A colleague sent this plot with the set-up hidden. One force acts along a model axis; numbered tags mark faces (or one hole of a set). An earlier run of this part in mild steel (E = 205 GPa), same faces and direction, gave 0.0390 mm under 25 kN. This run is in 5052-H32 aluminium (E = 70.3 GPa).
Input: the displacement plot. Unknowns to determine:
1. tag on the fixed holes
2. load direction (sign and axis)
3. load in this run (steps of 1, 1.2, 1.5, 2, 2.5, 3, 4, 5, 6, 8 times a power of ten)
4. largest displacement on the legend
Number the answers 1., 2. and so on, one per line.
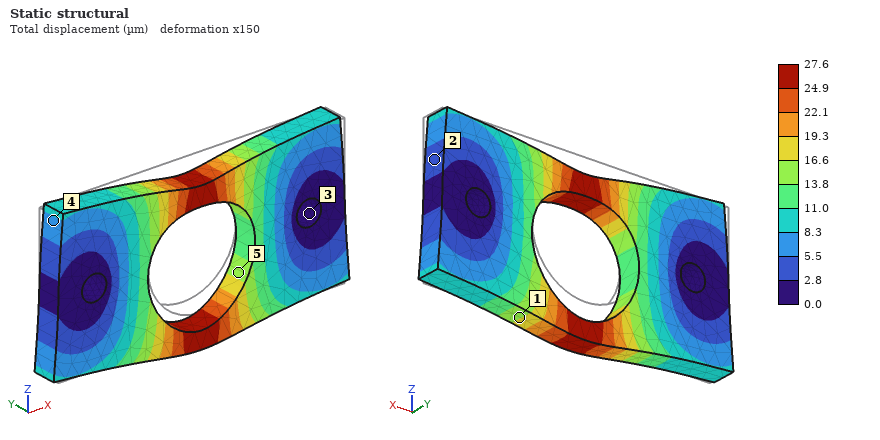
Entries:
1. 3
2. -Z
3. 6 kN
4. 27.6 µm
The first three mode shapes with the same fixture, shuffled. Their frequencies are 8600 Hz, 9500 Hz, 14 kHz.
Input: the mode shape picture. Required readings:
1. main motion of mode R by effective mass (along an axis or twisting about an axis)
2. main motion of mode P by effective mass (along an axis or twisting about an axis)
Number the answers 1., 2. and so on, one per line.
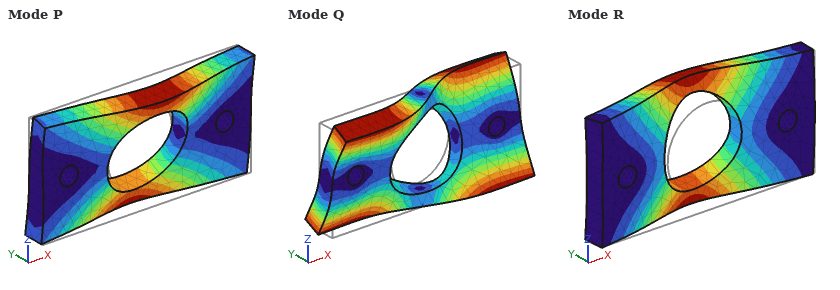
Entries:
1. along Y
2. twisting about X
